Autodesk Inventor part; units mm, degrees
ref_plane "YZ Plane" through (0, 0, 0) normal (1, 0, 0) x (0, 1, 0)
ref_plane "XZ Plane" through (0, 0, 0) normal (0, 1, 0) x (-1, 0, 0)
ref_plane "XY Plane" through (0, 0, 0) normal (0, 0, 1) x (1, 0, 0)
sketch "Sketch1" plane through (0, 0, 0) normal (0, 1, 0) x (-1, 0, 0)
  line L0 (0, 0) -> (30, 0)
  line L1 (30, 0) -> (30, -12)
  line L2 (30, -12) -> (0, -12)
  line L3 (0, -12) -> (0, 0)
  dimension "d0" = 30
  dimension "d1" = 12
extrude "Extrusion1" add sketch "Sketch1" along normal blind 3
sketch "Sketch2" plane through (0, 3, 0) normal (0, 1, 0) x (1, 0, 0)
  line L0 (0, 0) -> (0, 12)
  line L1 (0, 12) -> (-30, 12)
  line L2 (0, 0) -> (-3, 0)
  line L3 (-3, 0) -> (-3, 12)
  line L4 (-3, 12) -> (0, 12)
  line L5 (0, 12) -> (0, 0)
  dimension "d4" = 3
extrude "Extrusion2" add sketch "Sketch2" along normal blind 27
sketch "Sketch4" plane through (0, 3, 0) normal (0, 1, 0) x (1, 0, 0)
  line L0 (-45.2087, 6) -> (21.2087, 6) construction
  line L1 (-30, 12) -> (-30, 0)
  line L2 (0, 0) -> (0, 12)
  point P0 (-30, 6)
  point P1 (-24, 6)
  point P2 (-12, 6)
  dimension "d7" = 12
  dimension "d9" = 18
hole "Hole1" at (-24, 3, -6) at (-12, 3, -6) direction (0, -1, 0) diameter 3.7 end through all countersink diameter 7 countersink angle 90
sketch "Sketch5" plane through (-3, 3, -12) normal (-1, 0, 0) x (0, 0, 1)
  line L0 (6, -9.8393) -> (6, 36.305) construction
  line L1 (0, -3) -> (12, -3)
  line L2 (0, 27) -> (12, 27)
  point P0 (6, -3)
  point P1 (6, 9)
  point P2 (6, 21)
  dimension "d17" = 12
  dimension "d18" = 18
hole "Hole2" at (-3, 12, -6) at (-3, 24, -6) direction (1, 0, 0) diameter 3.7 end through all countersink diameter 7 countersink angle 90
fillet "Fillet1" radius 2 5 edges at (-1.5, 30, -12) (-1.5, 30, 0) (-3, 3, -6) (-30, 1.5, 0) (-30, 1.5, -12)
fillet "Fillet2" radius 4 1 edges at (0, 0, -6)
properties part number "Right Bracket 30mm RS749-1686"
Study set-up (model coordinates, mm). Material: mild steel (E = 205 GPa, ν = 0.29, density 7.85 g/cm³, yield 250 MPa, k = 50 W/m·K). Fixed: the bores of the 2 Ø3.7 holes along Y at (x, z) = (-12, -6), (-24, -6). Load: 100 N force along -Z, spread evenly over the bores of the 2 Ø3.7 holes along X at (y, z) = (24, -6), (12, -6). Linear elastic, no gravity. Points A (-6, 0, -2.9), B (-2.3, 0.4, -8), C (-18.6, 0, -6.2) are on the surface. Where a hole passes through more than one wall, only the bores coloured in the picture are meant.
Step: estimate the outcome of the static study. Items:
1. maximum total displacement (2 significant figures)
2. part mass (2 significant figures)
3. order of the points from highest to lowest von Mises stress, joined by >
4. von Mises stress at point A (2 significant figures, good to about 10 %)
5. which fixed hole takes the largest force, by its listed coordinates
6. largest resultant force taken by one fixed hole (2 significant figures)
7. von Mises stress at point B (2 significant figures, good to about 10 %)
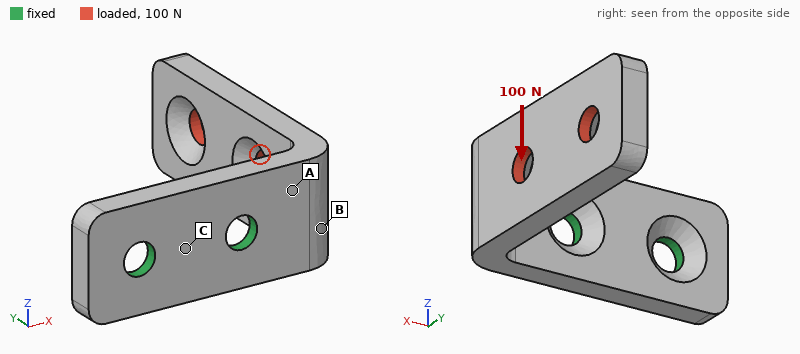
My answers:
74 µm
14 g
A > B > C
63 MPa
(-12, -6)
130 N
43 MPa
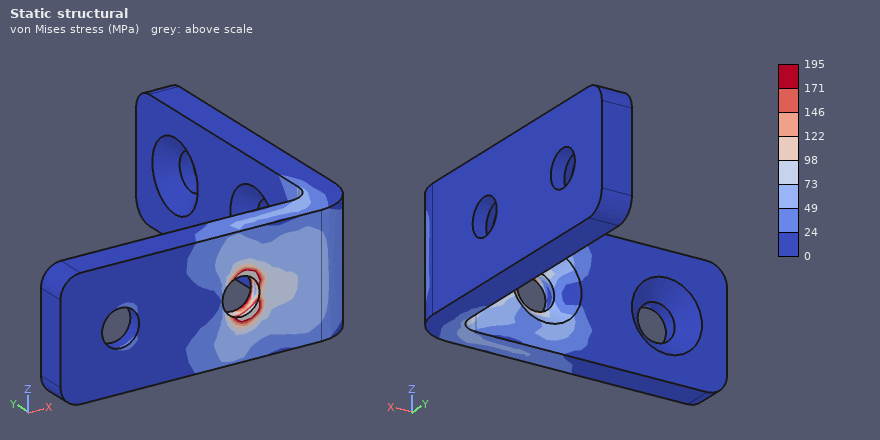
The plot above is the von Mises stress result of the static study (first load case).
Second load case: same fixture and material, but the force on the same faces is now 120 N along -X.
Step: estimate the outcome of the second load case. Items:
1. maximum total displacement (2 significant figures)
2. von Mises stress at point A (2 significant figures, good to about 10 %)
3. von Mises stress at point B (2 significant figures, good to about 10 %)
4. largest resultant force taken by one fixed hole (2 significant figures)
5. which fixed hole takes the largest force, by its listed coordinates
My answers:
0.19 mm
100 MPa
55 MPa
210 N
(-24, -6)
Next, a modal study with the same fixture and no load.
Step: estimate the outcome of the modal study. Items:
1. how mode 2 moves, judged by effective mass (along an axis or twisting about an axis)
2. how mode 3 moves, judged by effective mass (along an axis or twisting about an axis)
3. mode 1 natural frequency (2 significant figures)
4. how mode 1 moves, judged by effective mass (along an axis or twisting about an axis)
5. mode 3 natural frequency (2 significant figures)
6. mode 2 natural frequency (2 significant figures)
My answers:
along Z
along Y
2000 Hz
along X
7700 Hz
2800 Hz
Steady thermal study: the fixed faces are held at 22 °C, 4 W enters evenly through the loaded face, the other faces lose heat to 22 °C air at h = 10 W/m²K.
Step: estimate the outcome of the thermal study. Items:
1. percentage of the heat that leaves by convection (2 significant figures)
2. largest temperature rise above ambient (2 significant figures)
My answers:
10 %
61 K
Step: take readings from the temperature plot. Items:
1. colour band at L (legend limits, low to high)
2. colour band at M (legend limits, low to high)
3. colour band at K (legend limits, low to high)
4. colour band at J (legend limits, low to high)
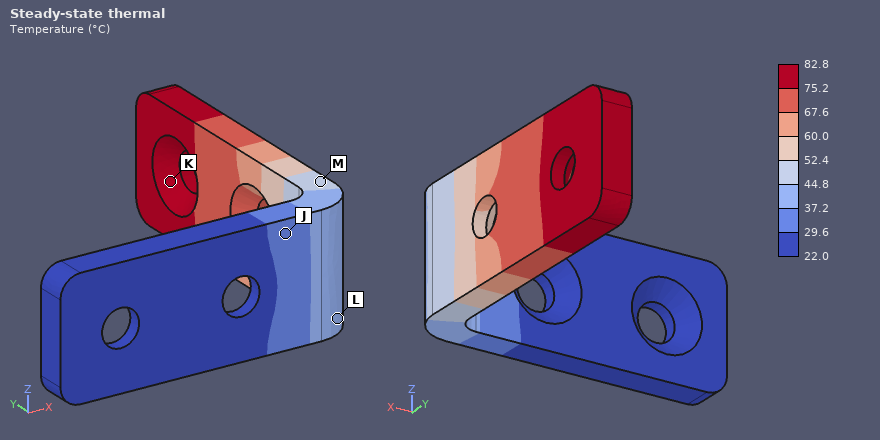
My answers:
37.2 to 44.8 °C
44.8 to 52.4 °C
75.2 to 82.8 °C
29.6 to 37.2 °C
